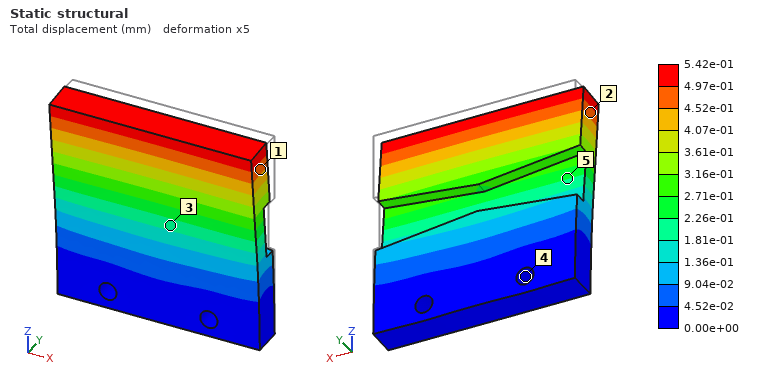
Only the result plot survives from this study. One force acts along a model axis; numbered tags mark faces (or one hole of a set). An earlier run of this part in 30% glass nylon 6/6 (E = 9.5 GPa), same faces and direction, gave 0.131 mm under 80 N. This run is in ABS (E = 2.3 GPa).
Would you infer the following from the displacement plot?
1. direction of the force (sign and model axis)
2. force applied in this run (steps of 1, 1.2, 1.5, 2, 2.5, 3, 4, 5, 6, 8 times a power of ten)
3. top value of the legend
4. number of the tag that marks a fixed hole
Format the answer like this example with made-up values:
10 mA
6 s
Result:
-Y
80 N
5.42e-01 mm
4
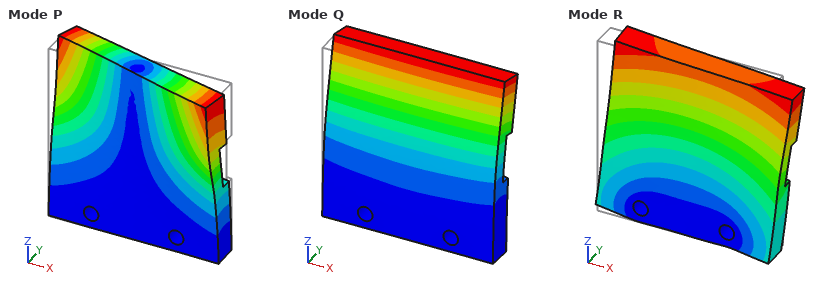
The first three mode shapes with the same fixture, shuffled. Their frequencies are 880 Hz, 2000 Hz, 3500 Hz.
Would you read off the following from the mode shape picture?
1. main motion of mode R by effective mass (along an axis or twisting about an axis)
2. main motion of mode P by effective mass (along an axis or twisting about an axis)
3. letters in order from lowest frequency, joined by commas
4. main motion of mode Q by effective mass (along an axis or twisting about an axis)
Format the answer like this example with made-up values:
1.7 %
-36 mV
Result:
along X
twisting about Z
Q, P, R
along Y
